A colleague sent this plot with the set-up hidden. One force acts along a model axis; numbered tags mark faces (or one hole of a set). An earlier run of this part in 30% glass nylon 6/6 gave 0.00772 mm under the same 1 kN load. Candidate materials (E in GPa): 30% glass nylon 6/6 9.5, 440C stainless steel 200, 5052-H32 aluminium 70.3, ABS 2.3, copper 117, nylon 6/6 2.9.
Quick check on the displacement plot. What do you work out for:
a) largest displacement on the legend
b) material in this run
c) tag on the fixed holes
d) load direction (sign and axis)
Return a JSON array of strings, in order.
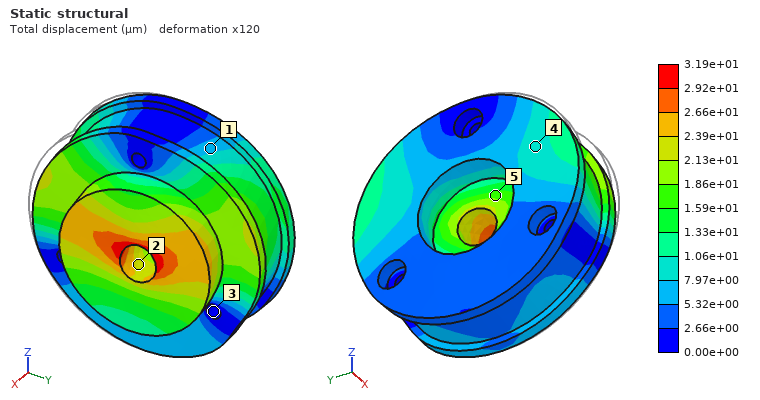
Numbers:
["3.19e+01 µm", "ABS", "3", "+Y"]
